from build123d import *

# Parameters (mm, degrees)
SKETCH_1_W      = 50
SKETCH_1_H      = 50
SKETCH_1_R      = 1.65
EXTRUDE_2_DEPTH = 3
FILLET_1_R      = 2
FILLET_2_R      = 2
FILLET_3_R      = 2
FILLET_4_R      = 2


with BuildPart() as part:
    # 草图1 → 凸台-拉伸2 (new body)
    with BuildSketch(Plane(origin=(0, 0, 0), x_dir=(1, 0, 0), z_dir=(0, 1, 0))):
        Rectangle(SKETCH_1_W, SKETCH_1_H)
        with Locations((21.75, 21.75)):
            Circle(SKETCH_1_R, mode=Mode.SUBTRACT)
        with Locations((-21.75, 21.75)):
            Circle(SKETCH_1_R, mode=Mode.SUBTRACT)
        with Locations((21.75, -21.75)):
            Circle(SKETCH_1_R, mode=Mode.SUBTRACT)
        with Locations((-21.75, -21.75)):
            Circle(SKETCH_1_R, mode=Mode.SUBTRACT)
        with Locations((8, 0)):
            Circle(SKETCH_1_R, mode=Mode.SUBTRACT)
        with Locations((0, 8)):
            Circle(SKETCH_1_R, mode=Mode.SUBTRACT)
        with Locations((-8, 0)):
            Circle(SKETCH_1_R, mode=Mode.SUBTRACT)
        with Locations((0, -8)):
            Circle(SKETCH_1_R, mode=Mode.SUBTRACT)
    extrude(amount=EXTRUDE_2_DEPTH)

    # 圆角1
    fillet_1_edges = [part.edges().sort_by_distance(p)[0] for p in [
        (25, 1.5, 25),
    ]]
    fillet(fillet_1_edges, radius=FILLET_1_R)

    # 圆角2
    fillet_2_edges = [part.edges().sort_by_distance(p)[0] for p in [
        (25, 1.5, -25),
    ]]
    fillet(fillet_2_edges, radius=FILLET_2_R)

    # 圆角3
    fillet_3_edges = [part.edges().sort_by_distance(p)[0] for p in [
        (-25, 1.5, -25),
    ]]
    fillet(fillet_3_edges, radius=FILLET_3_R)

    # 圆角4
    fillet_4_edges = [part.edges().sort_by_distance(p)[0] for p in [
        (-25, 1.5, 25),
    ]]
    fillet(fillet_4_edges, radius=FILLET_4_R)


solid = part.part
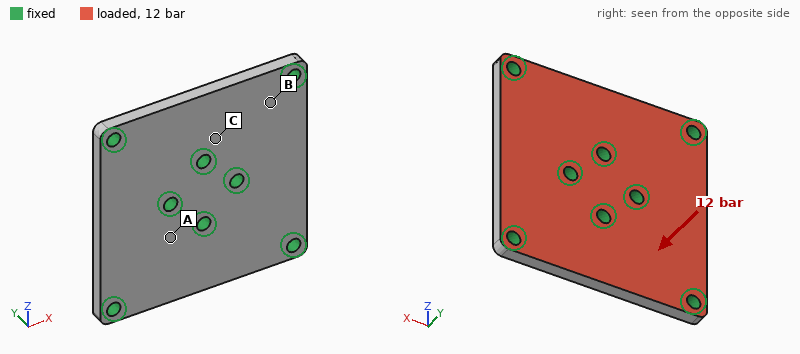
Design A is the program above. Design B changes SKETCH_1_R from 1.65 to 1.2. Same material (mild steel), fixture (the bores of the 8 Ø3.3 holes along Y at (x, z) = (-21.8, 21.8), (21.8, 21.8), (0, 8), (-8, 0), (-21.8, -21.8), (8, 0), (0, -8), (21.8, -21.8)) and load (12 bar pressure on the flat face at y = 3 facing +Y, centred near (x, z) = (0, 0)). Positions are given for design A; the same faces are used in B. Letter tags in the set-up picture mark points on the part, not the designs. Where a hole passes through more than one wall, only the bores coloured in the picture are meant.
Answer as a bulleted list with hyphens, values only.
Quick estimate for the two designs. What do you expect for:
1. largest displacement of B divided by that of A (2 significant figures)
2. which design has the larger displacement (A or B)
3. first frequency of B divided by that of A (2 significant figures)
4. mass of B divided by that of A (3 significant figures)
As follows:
- 1.1
- B
- 0.93
- 1.01
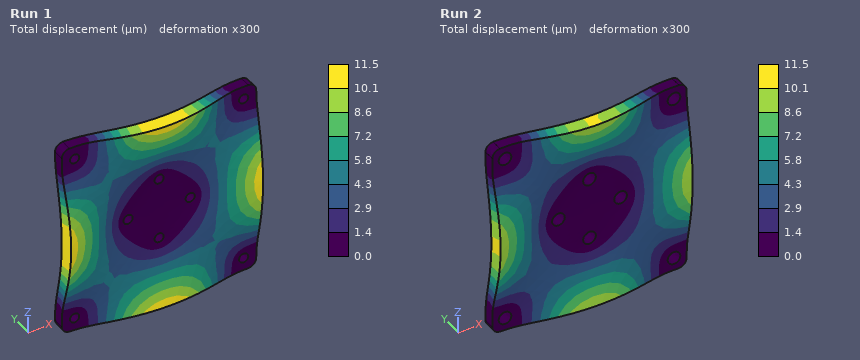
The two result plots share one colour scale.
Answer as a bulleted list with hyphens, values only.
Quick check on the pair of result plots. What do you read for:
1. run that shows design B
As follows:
- Run 1
